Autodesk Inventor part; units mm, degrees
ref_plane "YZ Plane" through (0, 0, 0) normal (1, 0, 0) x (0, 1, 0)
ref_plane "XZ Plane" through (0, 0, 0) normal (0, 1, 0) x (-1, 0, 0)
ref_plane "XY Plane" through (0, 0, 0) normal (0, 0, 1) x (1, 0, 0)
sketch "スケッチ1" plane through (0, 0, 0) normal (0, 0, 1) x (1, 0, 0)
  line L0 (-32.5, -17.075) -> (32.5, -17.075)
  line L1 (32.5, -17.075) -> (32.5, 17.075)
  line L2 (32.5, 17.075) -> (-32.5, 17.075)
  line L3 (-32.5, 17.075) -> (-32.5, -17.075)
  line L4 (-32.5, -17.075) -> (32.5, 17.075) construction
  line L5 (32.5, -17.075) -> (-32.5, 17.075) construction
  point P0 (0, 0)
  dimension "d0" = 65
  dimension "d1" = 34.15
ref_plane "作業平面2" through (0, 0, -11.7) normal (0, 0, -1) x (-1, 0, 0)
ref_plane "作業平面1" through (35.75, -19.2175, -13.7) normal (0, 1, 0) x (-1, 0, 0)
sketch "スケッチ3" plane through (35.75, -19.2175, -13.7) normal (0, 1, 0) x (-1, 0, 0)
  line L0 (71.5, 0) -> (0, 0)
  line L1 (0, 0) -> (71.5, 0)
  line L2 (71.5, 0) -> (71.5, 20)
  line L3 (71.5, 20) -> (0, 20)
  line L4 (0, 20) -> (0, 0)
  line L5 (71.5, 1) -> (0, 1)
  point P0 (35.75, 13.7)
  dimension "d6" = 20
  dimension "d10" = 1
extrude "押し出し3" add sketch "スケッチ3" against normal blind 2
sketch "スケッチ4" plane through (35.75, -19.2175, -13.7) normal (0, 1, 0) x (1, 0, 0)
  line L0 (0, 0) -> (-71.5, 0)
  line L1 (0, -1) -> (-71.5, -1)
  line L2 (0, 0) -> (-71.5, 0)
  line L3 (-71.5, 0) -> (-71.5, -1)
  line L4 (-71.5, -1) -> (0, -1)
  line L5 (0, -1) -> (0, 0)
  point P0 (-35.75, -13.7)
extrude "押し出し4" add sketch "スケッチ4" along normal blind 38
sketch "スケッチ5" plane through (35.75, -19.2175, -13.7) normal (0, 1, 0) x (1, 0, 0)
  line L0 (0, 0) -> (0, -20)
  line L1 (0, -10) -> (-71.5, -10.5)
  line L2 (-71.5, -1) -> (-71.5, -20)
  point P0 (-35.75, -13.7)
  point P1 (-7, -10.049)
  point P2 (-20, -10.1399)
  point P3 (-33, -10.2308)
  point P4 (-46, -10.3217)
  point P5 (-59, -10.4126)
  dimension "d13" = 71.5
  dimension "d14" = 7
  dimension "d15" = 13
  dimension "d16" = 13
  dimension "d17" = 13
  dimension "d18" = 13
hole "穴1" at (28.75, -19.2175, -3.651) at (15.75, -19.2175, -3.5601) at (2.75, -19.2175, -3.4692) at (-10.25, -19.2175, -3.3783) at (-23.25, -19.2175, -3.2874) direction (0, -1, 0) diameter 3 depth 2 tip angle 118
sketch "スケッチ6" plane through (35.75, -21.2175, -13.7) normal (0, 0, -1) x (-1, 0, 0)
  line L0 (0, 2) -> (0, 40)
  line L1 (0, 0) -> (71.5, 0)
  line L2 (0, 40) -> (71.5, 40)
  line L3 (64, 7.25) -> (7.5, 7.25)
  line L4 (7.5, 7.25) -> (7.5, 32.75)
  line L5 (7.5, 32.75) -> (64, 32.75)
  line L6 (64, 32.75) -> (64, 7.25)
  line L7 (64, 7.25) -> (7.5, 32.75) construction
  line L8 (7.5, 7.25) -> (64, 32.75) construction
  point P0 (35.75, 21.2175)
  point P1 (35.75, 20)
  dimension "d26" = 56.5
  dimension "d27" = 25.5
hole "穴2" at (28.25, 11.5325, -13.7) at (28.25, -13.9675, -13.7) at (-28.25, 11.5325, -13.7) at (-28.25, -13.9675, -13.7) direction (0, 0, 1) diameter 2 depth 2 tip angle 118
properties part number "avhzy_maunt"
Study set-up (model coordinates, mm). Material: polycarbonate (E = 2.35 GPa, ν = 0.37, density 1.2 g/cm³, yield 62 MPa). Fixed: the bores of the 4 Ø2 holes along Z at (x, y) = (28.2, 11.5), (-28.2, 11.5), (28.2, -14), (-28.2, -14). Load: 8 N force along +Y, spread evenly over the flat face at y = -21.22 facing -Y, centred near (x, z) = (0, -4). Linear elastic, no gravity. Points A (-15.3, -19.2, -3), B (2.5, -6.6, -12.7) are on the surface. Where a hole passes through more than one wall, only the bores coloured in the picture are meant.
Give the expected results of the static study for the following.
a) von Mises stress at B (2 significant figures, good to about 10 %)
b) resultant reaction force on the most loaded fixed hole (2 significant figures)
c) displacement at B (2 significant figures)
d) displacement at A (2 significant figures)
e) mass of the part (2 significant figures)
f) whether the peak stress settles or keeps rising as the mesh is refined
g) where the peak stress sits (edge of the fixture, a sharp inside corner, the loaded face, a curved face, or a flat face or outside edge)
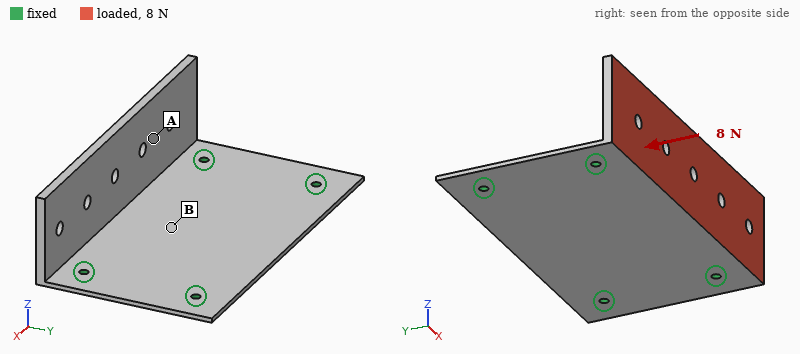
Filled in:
2.2 MPa
2.7 N
0.16 mm
0.44 mm
6.6 g
keeps rising
edge of the fixture
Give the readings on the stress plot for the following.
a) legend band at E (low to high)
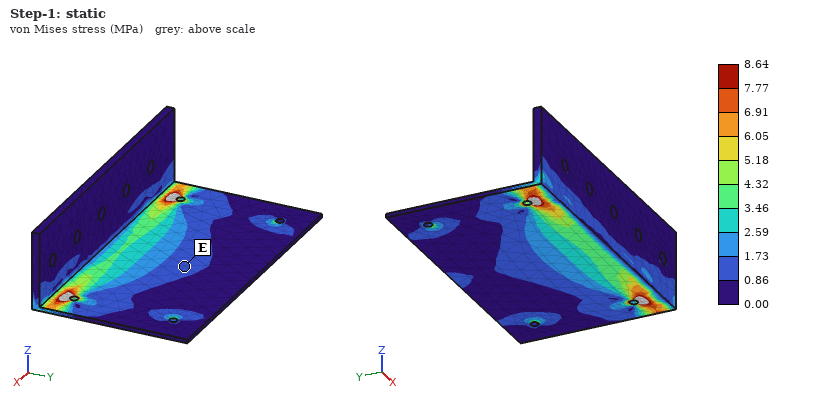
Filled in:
0.86 to 1.73 MPa
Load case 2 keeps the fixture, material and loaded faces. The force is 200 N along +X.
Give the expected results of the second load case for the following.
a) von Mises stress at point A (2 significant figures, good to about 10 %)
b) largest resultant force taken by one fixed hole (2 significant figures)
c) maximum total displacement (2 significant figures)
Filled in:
5.1 MPa
95 N
0.92 mm
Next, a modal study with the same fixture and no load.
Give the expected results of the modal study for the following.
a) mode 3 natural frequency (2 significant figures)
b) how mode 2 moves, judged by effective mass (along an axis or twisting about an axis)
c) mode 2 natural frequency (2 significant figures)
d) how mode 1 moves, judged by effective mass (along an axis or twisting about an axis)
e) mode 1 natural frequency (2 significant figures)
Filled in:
680 Hz
along Z
530 Hz
along Y
310 Hz
